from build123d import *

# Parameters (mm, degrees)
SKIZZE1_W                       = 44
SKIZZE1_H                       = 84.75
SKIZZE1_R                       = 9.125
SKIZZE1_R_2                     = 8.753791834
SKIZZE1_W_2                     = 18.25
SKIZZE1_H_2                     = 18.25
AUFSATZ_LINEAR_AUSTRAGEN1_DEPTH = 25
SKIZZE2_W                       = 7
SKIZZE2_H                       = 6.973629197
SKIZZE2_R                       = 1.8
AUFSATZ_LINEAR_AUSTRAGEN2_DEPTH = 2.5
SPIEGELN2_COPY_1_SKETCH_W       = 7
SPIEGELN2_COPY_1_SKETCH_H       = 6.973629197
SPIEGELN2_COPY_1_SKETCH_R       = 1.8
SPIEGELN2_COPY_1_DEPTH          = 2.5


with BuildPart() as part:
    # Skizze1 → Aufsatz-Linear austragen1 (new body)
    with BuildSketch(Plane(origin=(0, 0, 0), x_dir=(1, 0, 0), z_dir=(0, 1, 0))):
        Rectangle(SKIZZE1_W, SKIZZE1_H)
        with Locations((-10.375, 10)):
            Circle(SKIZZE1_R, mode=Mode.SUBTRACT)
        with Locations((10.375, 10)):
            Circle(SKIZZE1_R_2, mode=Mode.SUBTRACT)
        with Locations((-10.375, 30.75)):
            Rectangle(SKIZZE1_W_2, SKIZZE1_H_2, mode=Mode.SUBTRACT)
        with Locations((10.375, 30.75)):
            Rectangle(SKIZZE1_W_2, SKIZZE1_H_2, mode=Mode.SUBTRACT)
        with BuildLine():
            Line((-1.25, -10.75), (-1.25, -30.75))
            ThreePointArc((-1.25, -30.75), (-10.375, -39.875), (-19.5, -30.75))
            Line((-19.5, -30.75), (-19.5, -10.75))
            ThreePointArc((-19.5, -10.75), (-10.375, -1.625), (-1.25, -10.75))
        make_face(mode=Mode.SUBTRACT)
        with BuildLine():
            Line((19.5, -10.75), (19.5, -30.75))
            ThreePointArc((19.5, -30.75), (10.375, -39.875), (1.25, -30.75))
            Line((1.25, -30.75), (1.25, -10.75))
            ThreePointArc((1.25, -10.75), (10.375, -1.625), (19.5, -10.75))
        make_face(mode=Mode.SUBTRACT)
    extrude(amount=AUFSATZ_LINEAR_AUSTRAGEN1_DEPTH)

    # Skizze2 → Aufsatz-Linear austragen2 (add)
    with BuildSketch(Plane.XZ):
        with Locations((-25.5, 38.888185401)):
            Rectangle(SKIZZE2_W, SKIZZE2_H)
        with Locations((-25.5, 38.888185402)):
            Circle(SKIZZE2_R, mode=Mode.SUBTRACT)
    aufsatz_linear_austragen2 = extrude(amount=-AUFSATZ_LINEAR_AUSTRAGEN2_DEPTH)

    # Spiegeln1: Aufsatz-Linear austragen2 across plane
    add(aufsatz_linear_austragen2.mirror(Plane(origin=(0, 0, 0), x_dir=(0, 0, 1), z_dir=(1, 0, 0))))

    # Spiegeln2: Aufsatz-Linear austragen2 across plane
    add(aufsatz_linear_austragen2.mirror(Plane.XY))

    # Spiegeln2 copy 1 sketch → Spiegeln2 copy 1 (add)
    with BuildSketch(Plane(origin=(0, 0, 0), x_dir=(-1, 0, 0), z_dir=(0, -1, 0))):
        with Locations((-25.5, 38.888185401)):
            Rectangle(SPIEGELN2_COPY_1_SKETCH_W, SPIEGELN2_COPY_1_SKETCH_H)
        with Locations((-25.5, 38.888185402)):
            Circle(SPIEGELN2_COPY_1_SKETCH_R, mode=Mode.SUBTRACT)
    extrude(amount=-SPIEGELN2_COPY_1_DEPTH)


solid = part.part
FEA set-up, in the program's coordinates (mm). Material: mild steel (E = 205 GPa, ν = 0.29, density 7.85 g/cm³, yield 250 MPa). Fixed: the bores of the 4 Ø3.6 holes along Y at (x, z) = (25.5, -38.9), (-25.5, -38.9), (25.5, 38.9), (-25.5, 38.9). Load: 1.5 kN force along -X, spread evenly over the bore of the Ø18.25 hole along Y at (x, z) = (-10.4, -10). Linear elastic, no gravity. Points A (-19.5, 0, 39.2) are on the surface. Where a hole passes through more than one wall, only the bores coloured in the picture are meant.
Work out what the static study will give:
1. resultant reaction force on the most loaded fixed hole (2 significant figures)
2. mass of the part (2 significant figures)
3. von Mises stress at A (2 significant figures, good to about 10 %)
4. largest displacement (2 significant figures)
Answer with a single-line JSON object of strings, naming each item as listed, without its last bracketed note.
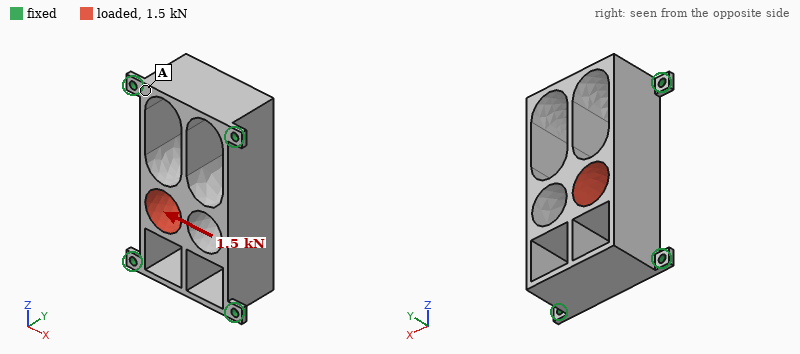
{"resultant reaction force on the most loaded fixed hole": "630 N", "mass of the part": "260 g", "von Mises stress at A": "17 MPa", "largest displacement": "45 µm"}
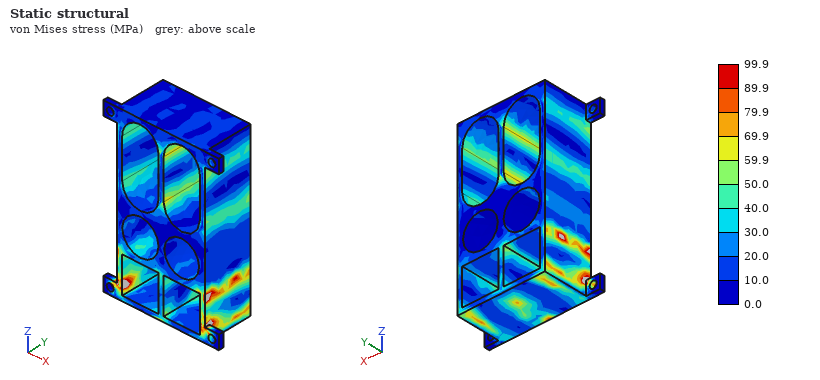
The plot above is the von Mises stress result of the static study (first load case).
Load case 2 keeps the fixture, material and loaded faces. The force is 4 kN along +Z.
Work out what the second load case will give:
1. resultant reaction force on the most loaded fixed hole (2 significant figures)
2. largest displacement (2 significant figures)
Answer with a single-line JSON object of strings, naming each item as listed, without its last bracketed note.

{"resultant reaction force on the most loaded fixed hole": "1.5 kN", "largest displacement": "18 µm"}
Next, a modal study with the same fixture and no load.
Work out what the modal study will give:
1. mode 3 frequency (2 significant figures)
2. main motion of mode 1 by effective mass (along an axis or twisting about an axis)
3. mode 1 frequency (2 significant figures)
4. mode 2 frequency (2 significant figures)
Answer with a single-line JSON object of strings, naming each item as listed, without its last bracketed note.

{"mode 3 frequency": "5700 Hz", "main motion of mode 1 by effective mass": "along X", "mode 1 frequency": "2500 Hz", "mode 2 frequency": "5600 Hz"}
